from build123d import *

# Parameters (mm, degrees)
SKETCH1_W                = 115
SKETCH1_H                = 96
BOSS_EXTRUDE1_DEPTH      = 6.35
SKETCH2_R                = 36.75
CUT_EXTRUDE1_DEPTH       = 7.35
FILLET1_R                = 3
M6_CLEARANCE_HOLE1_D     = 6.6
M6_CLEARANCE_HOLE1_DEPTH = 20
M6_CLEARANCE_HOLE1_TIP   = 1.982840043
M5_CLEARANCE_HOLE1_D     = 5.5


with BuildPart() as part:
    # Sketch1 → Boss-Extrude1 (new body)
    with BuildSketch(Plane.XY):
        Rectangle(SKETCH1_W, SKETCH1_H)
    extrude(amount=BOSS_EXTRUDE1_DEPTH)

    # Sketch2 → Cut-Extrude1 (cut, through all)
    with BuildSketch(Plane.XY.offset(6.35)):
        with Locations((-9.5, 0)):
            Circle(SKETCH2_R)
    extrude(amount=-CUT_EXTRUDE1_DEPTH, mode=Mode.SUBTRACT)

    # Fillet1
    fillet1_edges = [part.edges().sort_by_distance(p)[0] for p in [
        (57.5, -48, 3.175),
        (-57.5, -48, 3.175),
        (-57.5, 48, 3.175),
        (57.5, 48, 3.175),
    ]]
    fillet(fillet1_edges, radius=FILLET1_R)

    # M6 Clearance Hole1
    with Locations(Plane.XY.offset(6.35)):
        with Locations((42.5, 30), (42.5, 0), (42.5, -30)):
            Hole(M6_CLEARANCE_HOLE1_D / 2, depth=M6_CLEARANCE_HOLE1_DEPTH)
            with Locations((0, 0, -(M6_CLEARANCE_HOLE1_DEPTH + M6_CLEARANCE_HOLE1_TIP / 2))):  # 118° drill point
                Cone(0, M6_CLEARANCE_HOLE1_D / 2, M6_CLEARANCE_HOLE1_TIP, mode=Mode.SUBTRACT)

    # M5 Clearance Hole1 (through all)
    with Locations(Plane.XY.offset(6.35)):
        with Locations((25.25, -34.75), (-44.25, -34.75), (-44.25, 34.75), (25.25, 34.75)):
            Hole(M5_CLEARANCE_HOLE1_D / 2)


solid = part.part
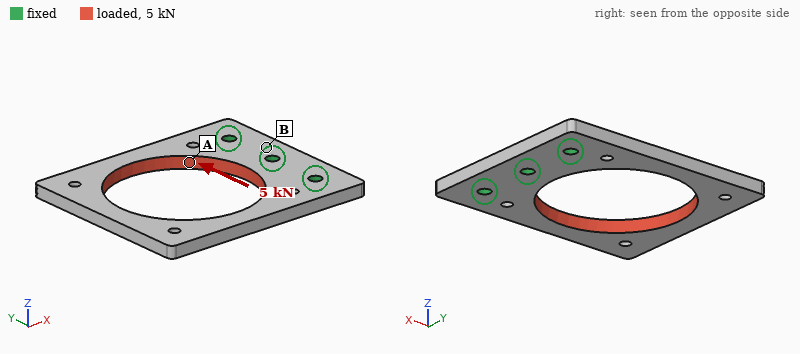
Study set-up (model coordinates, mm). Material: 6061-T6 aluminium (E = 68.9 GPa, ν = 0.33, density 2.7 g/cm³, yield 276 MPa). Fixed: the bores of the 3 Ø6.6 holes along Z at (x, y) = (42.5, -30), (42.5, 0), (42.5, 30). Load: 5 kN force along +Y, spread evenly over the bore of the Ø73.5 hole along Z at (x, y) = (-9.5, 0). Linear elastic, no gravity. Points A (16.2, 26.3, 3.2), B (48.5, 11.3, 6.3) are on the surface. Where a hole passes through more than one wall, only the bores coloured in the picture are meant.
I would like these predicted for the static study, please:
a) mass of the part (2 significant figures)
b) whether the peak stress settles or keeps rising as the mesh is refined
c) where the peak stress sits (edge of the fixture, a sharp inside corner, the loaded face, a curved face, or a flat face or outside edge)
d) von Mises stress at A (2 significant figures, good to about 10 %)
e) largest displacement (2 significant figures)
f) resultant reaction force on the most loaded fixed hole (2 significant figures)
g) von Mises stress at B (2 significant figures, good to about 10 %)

110 g
keeps rising
edge of the fixture
110 MPa
0.36 mm
3.8 kN
15 MPa
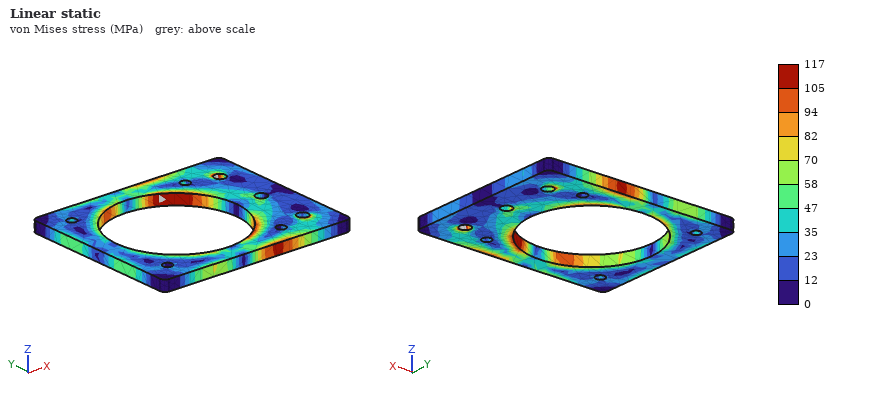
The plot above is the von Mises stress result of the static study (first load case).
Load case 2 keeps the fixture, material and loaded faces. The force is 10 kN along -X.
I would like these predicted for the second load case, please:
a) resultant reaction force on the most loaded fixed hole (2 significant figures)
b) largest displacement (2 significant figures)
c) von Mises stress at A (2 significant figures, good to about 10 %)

5.5 kN
0.16 mm
32 MPa
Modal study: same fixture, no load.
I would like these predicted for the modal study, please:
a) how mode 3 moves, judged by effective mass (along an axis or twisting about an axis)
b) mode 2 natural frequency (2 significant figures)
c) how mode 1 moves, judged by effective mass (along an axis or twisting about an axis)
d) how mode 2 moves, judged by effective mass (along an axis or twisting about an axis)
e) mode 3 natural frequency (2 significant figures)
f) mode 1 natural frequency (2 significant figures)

along Y
960 Hz
along Z
twisting about X
2200 Hz
420 Hz
